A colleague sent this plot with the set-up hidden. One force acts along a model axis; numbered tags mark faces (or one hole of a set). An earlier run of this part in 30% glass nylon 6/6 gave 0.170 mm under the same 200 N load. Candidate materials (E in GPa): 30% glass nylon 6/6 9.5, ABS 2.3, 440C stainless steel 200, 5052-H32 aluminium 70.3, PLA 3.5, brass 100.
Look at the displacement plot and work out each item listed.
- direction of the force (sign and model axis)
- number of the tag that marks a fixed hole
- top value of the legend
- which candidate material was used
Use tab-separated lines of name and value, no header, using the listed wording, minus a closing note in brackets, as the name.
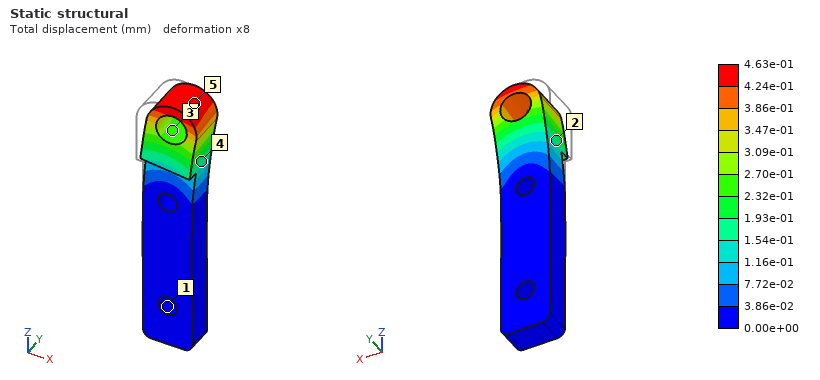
direction of the force	+X
number of the tag that marks a fixed hole	1
top value of the legend	4.63e-01 mm
which candidate material was used	PLA
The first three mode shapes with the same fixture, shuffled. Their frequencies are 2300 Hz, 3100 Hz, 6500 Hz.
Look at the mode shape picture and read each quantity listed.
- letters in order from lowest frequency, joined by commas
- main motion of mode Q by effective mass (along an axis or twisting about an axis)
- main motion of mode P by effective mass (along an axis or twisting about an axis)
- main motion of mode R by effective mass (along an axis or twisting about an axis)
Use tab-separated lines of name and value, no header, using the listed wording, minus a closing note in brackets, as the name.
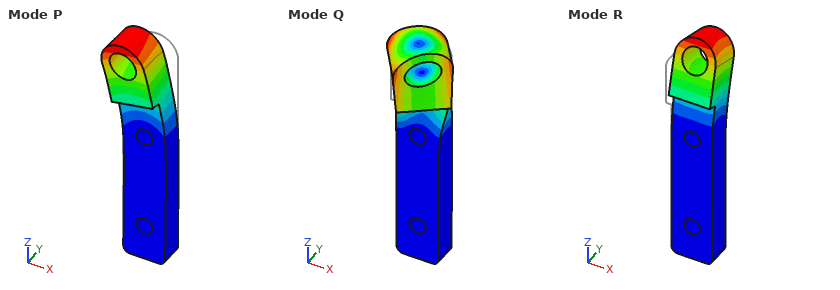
letters in order from lowest frequency, joined by commas	R, P, Q
main motion of mode Q by effective mass	twisting about Z
main motion of mode P by effective mass	along X
main motion of mode R by effective mass	along Y
